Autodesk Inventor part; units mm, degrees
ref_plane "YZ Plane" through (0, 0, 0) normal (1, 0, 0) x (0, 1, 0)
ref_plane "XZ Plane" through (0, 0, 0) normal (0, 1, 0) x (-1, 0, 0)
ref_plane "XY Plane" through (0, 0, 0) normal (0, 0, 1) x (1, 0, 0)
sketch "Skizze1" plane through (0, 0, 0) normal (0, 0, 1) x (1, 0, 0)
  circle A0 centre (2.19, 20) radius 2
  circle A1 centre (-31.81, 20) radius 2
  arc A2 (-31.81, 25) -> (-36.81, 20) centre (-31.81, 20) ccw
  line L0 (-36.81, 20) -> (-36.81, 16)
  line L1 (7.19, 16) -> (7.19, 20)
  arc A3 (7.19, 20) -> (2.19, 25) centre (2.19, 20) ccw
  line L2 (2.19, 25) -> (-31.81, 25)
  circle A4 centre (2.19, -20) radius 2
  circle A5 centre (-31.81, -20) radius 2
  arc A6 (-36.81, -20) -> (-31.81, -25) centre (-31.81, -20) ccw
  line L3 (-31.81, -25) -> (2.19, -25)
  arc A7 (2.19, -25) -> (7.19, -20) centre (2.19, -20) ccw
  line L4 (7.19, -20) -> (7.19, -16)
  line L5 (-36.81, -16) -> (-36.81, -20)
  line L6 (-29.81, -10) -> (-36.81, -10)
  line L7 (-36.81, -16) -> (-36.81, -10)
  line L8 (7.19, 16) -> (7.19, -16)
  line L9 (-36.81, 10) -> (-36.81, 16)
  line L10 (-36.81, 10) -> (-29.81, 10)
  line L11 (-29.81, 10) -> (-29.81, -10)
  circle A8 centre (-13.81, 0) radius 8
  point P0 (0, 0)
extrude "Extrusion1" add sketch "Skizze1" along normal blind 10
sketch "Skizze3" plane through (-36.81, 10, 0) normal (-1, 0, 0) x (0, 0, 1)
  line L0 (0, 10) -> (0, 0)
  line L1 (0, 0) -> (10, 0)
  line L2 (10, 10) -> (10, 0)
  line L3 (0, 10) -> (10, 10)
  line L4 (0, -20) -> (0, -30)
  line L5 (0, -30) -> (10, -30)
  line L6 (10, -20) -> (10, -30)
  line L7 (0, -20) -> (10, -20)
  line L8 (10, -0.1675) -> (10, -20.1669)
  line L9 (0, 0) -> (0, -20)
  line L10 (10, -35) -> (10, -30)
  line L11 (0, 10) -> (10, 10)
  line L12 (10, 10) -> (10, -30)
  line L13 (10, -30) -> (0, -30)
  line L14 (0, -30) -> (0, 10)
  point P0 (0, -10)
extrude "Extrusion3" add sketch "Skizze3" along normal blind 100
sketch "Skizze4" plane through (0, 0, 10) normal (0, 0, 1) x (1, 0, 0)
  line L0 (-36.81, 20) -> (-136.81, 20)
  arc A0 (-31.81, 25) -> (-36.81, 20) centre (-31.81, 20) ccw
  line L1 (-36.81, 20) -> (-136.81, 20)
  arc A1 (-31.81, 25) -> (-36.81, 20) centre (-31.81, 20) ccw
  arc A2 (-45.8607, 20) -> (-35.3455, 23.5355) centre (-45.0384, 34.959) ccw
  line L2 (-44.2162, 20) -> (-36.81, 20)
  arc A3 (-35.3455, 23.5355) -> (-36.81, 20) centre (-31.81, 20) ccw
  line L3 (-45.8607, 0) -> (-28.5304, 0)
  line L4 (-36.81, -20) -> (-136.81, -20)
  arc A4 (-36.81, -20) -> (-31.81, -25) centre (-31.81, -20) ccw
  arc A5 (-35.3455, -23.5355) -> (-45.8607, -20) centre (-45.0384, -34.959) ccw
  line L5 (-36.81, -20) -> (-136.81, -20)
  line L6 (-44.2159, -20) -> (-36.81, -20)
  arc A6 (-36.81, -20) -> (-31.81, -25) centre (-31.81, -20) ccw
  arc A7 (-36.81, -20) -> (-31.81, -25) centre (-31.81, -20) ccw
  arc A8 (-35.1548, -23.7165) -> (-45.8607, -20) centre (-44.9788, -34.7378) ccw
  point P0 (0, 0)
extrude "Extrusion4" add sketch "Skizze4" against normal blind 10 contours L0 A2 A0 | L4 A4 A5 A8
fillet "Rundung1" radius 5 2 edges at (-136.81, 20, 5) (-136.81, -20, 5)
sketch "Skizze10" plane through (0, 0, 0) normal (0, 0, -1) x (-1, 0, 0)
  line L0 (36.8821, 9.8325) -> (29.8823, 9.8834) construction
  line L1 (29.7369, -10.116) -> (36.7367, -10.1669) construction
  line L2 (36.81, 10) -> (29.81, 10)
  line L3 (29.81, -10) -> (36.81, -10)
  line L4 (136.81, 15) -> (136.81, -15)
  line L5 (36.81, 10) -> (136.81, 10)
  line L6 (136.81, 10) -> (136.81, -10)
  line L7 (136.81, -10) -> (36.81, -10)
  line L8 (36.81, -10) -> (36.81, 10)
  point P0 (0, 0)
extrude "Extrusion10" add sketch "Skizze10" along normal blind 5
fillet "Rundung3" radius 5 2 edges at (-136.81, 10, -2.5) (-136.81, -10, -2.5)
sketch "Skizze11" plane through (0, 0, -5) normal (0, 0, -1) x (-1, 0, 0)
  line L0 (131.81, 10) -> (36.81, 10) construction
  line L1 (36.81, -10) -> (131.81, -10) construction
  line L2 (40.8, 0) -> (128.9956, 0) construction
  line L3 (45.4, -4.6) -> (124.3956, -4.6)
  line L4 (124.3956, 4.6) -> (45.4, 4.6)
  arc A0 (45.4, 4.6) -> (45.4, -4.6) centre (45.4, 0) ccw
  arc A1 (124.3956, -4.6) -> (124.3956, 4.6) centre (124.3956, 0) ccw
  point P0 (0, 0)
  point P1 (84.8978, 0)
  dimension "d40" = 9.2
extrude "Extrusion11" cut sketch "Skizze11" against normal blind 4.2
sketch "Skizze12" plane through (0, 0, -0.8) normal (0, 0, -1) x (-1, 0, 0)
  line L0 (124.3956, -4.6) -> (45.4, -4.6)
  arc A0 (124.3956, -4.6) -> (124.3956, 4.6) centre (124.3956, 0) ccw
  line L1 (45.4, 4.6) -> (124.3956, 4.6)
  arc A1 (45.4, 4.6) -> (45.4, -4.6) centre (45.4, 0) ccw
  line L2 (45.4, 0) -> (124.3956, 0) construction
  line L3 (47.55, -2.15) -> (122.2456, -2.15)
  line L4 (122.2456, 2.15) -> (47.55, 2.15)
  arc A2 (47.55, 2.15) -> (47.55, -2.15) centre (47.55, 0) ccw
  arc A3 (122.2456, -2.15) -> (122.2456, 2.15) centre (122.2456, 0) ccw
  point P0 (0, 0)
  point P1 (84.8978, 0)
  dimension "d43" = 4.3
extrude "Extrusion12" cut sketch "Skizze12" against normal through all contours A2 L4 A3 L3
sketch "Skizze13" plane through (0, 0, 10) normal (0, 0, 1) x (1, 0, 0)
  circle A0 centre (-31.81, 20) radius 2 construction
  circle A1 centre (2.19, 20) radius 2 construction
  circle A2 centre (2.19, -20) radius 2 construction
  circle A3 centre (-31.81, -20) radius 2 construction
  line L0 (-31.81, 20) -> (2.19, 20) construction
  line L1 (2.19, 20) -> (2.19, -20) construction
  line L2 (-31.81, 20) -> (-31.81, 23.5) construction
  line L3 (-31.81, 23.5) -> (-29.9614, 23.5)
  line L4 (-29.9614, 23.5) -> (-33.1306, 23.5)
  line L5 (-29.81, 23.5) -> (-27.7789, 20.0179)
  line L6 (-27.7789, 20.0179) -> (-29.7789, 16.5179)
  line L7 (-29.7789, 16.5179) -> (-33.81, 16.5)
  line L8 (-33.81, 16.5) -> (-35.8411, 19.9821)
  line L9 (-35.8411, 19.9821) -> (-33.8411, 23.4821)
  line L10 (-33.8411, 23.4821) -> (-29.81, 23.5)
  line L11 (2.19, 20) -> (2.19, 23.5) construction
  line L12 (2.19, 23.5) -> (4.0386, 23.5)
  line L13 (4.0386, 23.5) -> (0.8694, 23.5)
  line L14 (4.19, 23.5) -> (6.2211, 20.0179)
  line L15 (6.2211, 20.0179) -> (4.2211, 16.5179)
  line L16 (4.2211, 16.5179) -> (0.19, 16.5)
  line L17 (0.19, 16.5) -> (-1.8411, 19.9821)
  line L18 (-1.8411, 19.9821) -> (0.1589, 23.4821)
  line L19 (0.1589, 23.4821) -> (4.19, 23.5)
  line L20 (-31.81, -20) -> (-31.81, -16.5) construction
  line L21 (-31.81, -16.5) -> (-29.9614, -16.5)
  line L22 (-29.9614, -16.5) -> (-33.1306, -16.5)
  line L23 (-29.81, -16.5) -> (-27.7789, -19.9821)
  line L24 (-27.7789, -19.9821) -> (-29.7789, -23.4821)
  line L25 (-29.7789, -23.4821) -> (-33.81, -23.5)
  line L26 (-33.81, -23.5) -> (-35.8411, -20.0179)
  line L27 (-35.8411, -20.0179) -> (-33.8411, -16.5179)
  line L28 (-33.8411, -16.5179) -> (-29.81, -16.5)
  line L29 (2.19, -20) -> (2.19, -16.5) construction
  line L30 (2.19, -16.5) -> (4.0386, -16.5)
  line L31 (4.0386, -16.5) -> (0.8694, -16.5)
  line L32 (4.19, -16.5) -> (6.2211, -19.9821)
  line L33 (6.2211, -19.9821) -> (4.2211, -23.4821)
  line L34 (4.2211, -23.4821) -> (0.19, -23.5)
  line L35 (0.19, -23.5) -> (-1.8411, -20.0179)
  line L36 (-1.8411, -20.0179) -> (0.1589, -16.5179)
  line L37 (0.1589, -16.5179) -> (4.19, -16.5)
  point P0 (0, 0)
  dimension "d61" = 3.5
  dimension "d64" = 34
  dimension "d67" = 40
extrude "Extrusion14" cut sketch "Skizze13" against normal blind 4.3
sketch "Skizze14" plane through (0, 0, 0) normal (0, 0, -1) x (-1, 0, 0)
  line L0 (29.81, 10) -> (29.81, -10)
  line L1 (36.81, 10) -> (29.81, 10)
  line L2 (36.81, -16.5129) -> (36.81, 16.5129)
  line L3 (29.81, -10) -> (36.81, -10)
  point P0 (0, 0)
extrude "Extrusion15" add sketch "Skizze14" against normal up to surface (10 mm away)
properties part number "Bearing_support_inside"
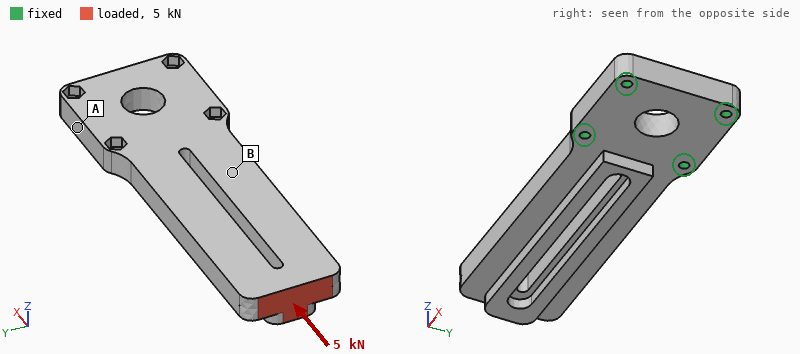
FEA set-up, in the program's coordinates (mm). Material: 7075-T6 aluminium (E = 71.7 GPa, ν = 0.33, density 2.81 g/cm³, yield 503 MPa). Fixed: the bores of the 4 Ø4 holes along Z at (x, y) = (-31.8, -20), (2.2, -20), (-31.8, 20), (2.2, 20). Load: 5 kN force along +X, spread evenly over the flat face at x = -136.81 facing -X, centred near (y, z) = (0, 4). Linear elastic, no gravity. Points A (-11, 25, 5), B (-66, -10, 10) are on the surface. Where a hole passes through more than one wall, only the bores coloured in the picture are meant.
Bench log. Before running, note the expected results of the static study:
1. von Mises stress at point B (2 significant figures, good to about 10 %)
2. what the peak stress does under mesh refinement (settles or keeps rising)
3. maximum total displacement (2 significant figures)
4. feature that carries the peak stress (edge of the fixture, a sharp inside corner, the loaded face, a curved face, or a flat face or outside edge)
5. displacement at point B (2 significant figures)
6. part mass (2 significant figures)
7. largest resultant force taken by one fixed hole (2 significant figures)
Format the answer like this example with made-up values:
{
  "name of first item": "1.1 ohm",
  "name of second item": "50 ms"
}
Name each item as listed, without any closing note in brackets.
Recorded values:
{
  "von Mises stress at point B": "12 MPa",
  "what the peak stress does under mesh refinement": "keeps rising",
  "maximum total displacement": "27 µm",
  "feature that carries the peak stress": "edge of the fixture",
  "displacement at point B": "7.9 µm",
  "part mass": "170 g",
  "largest resultant force taken by one fixed hole": "2.0 kN"
}
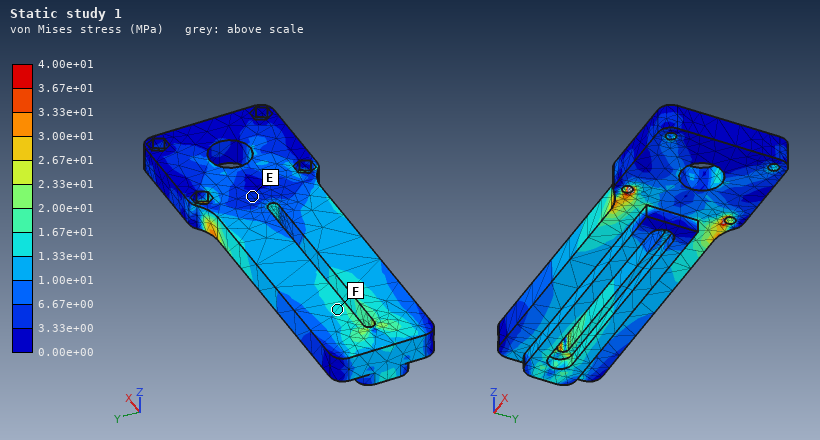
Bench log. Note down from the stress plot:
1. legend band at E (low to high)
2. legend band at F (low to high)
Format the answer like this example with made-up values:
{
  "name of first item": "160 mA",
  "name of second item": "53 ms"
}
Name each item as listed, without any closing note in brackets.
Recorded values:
{
  "legend band at E": "3.33e+00 to 6.67e+00 MPa",
  "legend band at F": "1.33e+01 to 1.67e+01 MPa"
}
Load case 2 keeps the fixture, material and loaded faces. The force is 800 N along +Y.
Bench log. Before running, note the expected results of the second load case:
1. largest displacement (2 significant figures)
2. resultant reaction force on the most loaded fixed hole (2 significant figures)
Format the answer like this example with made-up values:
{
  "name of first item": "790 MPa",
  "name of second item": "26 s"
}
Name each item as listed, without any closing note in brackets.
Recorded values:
{
  "largest displacement": "0.14 mm",
  "resultant reaction force on the most loaded fixed hole": "1.9 kN"
}
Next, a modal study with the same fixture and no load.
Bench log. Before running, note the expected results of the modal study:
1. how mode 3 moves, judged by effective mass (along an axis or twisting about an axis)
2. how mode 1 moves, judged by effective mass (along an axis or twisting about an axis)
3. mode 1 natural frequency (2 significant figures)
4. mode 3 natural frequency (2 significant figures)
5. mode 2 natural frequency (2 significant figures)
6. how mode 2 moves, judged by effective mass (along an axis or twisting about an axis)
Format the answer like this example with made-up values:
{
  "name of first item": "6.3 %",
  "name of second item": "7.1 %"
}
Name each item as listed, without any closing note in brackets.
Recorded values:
{
  "how mode 3 moves, judged by effective mass": "twisting about X",
  "how mode 1 moves, judged by effective mass": "along Z",
  "mode 1 natural frequency": "700 Hz",
  "mode 3 natural frequency": "3100 Hz",
  "mode 2 natural frequency": "1900 Hz",
  "how mode 2 moves, judged by effective mass": "along Y"
}
